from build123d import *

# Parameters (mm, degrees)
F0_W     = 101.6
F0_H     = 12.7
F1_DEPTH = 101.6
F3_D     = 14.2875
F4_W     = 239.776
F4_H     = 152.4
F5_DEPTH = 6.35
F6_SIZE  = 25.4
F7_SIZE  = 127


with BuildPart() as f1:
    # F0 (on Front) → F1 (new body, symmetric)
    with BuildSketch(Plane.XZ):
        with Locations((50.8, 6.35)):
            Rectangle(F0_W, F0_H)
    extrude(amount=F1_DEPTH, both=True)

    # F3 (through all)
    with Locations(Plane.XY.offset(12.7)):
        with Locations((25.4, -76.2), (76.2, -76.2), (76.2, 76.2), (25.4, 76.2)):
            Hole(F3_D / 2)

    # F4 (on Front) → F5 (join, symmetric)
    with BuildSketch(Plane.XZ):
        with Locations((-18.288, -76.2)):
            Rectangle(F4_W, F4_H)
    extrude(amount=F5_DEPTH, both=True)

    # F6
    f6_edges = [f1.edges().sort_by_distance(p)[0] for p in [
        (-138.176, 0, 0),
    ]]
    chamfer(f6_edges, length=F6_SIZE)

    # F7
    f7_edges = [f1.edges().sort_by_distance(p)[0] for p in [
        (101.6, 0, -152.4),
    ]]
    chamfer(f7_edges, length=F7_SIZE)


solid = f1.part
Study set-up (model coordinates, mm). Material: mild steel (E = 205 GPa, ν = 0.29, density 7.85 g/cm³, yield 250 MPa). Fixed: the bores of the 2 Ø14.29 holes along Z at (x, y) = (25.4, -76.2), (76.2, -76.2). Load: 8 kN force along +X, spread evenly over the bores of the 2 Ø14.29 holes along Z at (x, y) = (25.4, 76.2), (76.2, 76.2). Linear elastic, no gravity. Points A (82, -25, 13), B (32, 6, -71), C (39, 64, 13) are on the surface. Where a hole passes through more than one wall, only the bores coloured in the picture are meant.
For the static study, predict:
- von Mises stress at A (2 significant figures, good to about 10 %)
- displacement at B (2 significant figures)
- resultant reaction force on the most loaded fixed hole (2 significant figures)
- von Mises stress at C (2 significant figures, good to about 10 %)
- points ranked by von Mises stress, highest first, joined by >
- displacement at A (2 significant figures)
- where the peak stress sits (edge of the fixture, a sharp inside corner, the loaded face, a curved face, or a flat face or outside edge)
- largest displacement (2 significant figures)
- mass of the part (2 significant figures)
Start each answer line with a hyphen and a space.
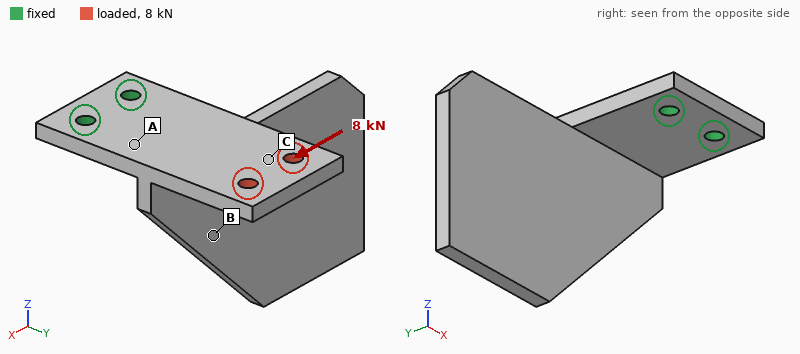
- 25 MPa
- 25 µm
- 20 kN
- 13 MPa
- A > C > B
- 17 µm
- edge of the fixture
- 81 µm
- 4.8 kg
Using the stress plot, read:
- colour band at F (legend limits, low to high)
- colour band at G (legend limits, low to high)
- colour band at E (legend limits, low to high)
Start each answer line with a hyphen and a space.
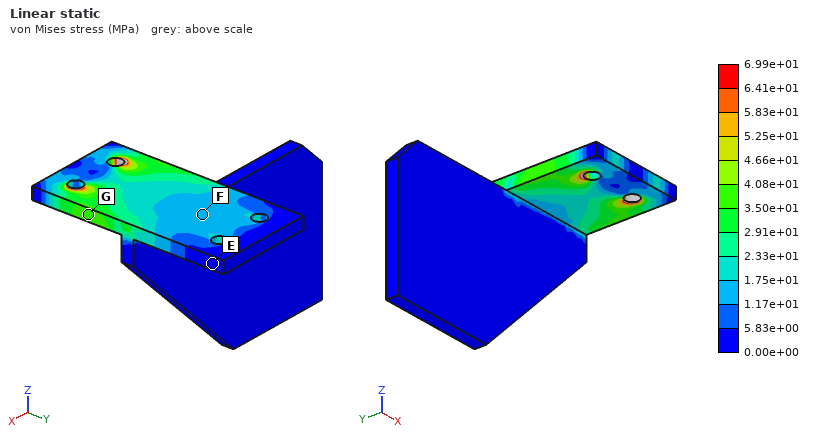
- 1.17e+01 to 1.75e+01 MPa
- 3.50e+01 to 4.08e+01 MPa
- 0.00e+00 to 5.83e+00 MPa
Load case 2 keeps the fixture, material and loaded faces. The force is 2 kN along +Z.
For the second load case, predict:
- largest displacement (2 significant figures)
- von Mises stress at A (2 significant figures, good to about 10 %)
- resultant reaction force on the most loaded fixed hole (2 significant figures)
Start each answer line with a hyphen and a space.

- 0.75 mm
- 69 MPa
- 1.0 kN
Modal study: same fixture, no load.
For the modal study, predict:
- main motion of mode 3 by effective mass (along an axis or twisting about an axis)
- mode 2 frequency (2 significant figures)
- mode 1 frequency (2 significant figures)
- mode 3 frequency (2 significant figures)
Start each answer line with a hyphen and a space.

- along Z
- 250 Hz
- 150 Hz
- 380 Hz
